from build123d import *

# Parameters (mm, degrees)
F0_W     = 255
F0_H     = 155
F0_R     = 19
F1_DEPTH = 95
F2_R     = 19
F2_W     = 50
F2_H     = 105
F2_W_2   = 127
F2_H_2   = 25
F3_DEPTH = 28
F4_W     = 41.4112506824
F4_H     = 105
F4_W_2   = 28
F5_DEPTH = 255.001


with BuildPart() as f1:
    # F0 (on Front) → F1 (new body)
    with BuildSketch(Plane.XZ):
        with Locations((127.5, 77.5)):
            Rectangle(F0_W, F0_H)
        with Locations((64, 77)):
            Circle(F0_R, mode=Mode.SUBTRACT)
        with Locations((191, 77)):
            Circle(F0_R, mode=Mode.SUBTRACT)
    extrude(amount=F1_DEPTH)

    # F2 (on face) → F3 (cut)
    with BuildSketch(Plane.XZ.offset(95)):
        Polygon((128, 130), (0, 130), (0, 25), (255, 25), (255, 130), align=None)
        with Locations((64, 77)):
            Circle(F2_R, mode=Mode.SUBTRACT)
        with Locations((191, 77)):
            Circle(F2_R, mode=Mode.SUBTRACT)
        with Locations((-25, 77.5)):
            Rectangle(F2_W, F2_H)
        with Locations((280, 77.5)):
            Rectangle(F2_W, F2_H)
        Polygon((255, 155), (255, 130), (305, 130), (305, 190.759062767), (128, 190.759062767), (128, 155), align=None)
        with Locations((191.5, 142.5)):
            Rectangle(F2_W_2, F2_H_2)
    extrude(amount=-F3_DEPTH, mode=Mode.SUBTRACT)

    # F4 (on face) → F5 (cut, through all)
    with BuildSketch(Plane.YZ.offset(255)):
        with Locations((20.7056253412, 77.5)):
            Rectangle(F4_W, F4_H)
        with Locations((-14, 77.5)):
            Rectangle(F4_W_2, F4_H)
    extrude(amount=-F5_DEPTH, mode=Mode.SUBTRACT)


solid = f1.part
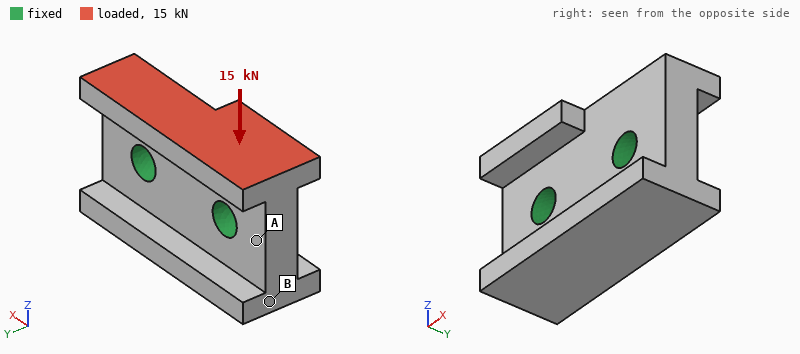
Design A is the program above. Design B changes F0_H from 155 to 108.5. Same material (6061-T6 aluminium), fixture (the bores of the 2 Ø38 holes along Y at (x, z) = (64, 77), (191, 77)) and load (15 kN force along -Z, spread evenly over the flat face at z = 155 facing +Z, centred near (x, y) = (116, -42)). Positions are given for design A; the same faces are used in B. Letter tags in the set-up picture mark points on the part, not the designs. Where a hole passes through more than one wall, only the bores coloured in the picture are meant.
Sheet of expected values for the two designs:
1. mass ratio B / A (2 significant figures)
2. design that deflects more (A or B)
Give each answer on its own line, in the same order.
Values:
0.50
B
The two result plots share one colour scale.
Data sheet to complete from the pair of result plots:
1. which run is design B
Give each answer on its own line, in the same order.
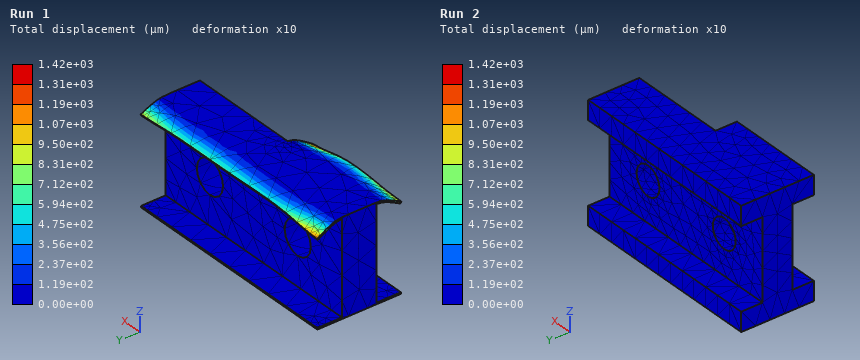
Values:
Run 1
